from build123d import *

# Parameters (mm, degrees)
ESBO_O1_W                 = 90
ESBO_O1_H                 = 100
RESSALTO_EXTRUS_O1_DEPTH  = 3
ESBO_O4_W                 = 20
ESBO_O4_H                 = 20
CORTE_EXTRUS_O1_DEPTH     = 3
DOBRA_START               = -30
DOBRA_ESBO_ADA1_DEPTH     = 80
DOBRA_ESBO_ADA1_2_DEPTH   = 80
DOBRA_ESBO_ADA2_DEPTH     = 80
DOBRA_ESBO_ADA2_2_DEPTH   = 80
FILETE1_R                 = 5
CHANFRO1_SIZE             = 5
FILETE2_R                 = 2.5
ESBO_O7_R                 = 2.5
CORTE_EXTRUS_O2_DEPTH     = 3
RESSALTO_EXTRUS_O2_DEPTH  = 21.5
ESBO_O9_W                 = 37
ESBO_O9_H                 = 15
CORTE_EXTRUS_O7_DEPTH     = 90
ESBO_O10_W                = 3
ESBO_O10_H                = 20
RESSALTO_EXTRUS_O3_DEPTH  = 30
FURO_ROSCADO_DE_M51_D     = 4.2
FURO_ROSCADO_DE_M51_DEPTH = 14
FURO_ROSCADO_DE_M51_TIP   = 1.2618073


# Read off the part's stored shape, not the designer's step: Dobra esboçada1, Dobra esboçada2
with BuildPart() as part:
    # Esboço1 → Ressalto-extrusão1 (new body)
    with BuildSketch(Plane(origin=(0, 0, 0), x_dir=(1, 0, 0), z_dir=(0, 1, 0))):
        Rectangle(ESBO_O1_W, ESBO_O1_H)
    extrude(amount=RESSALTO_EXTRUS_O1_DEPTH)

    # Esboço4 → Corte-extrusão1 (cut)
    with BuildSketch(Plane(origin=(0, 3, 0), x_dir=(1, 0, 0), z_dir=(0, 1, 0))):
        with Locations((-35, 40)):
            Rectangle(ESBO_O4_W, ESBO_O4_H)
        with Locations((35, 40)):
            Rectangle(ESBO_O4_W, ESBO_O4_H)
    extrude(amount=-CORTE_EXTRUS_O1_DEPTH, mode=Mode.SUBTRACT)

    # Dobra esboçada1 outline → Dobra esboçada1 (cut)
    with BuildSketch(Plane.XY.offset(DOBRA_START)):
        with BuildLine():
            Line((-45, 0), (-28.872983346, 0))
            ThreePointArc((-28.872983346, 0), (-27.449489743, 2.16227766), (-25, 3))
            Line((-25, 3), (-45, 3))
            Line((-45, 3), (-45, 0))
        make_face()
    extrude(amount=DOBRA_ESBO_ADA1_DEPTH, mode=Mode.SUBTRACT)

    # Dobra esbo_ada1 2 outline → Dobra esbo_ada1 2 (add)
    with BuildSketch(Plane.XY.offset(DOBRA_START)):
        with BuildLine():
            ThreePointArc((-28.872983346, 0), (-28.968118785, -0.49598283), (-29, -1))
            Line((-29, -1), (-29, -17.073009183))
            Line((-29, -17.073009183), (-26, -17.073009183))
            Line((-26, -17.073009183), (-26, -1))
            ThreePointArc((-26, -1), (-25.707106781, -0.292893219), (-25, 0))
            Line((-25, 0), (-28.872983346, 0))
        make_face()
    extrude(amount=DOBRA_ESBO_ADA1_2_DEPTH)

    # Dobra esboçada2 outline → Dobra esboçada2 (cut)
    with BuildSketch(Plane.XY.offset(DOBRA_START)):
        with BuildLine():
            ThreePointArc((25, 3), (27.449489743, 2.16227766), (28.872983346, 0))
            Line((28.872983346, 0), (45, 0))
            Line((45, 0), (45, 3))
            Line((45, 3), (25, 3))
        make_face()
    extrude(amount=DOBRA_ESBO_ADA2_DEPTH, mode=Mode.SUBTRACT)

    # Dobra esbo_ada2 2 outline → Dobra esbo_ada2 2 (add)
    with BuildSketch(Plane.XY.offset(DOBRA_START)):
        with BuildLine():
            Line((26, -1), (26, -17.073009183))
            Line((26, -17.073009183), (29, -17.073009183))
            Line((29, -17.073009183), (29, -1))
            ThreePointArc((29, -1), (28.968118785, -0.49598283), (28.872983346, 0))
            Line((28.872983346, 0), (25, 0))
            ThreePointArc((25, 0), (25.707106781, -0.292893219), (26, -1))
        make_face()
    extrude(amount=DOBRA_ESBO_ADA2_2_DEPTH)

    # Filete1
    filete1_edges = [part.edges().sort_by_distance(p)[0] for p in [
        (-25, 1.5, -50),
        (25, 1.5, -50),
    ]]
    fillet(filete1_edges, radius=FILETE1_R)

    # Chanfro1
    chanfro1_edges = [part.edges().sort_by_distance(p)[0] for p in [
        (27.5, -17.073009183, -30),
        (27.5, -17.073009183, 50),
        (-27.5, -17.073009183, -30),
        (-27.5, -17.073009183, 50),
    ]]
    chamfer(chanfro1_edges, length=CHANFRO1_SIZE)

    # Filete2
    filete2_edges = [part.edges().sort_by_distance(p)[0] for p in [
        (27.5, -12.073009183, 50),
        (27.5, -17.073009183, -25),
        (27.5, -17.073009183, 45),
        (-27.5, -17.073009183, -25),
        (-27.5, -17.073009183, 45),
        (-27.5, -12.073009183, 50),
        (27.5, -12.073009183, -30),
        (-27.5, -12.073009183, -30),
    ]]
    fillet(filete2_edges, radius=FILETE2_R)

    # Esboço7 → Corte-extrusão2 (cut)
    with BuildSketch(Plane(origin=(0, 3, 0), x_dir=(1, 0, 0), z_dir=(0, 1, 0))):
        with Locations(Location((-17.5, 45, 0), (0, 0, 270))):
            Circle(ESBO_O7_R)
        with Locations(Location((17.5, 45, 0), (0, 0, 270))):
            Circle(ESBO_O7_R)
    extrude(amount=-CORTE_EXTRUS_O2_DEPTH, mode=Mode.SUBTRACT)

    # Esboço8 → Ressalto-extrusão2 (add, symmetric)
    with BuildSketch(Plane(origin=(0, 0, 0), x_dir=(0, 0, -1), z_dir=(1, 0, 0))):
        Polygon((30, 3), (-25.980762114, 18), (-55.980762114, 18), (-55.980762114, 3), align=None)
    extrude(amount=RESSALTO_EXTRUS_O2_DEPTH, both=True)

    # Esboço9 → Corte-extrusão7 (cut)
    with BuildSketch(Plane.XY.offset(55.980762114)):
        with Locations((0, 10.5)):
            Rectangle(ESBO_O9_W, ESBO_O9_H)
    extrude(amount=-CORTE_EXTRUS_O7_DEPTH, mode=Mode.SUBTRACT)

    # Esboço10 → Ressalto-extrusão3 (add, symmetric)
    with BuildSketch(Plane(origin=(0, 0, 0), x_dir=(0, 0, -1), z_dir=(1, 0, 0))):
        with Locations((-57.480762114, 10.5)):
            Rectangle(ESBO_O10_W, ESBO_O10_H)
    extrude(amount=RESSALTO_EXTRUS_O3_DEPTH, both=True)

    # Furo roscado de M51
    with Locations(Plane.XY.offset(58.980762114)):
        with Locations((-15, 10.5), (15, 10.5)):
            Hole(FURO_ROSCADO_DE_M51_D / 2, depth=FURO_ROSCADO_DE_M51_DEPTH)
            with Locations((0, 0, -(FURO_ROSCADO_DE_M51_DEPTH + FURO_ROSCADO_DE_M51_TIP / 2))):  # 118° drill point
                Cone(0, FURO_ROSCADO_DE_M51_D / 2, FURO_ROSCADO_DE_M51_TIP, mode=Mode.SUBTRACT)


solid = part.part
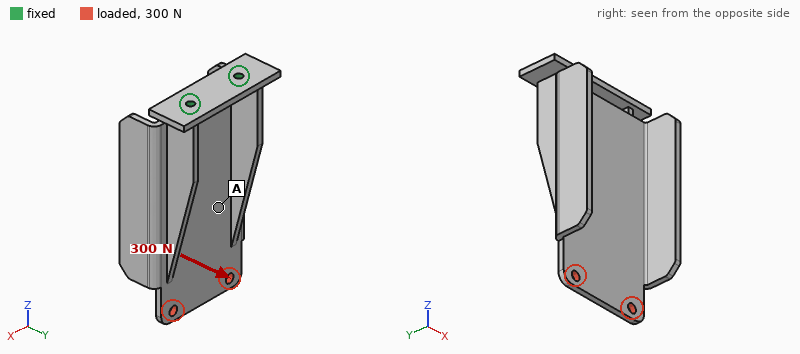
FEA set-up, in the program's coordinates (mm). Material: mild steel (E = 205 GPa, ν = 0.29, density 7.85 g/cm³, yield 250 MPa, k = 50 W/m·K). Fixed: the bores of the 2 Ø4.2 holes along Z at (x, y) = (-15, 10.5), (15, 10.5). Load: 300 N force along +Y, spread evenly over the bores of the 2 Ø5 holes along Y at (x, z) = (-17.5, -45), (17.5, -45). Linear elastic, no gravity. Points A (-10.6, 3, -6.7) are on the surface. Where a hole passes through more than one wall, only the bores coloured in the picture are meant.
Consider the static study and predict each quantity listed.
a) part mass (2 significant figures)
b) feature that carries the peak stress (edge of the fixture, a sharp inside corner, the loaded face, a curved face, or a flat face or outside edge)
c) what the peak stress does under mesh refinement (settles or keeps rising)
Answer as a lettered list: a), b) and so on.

a) 260 g
b) edge of the fixture
c) keeps rising
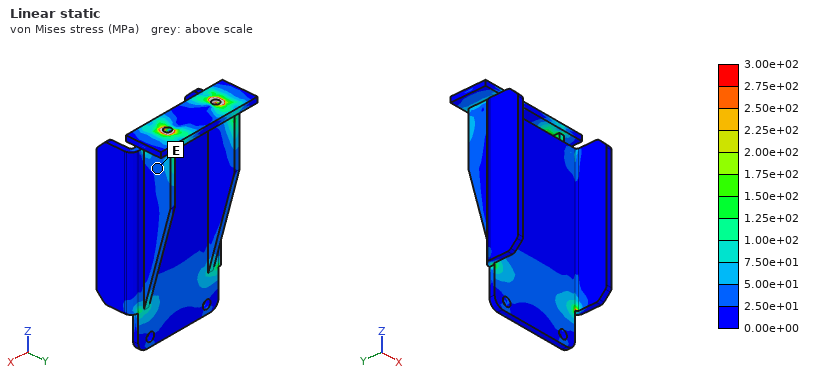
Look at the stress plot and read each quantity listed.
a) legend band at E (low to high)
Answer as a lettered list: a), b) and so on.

a) 2.50e+01 to 5.00e+01 MPa
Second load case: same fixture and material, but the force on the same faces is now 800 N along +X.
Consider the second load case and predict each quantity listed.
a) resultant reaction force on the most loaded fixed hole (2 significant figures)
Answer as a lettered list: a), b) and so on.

a) 2.1 kN
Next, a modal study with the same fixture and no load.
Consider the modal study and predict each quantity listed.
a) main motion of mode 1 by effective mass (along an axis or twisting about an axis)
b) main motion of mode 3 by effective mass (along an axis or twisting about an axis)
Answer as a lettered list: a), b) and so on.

a) along Y
b) along X
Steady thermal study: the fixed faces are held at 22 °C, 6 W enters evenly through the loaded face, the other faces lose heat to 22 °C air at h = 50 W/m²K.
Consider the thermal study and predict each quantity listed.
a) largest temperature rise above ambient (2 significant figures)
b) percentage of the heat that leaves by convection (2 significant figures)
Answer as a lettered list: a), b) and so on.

a) 28 K
b) 94 %
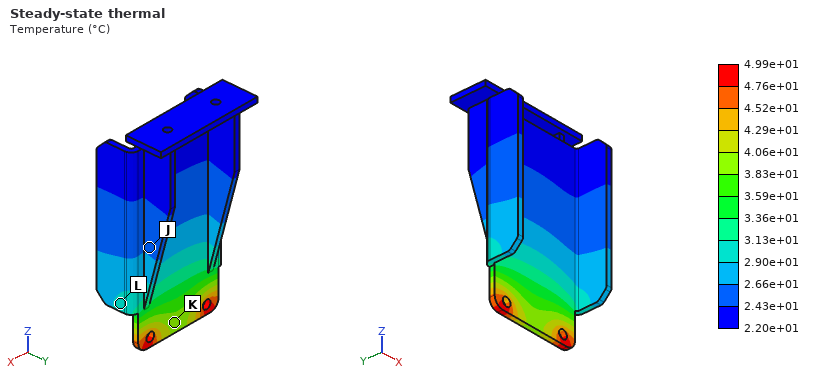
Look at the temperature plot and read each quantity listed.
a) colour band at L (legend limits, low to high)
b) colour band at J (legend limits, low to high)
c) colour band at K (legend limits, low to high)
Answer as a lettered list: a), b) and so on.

a) 2.90e+01 to 3.13e+01 °C
b) 2.43e+01 to 2.66e+01 °C
c) 3.83e+01 to 4.06e+01 °C
